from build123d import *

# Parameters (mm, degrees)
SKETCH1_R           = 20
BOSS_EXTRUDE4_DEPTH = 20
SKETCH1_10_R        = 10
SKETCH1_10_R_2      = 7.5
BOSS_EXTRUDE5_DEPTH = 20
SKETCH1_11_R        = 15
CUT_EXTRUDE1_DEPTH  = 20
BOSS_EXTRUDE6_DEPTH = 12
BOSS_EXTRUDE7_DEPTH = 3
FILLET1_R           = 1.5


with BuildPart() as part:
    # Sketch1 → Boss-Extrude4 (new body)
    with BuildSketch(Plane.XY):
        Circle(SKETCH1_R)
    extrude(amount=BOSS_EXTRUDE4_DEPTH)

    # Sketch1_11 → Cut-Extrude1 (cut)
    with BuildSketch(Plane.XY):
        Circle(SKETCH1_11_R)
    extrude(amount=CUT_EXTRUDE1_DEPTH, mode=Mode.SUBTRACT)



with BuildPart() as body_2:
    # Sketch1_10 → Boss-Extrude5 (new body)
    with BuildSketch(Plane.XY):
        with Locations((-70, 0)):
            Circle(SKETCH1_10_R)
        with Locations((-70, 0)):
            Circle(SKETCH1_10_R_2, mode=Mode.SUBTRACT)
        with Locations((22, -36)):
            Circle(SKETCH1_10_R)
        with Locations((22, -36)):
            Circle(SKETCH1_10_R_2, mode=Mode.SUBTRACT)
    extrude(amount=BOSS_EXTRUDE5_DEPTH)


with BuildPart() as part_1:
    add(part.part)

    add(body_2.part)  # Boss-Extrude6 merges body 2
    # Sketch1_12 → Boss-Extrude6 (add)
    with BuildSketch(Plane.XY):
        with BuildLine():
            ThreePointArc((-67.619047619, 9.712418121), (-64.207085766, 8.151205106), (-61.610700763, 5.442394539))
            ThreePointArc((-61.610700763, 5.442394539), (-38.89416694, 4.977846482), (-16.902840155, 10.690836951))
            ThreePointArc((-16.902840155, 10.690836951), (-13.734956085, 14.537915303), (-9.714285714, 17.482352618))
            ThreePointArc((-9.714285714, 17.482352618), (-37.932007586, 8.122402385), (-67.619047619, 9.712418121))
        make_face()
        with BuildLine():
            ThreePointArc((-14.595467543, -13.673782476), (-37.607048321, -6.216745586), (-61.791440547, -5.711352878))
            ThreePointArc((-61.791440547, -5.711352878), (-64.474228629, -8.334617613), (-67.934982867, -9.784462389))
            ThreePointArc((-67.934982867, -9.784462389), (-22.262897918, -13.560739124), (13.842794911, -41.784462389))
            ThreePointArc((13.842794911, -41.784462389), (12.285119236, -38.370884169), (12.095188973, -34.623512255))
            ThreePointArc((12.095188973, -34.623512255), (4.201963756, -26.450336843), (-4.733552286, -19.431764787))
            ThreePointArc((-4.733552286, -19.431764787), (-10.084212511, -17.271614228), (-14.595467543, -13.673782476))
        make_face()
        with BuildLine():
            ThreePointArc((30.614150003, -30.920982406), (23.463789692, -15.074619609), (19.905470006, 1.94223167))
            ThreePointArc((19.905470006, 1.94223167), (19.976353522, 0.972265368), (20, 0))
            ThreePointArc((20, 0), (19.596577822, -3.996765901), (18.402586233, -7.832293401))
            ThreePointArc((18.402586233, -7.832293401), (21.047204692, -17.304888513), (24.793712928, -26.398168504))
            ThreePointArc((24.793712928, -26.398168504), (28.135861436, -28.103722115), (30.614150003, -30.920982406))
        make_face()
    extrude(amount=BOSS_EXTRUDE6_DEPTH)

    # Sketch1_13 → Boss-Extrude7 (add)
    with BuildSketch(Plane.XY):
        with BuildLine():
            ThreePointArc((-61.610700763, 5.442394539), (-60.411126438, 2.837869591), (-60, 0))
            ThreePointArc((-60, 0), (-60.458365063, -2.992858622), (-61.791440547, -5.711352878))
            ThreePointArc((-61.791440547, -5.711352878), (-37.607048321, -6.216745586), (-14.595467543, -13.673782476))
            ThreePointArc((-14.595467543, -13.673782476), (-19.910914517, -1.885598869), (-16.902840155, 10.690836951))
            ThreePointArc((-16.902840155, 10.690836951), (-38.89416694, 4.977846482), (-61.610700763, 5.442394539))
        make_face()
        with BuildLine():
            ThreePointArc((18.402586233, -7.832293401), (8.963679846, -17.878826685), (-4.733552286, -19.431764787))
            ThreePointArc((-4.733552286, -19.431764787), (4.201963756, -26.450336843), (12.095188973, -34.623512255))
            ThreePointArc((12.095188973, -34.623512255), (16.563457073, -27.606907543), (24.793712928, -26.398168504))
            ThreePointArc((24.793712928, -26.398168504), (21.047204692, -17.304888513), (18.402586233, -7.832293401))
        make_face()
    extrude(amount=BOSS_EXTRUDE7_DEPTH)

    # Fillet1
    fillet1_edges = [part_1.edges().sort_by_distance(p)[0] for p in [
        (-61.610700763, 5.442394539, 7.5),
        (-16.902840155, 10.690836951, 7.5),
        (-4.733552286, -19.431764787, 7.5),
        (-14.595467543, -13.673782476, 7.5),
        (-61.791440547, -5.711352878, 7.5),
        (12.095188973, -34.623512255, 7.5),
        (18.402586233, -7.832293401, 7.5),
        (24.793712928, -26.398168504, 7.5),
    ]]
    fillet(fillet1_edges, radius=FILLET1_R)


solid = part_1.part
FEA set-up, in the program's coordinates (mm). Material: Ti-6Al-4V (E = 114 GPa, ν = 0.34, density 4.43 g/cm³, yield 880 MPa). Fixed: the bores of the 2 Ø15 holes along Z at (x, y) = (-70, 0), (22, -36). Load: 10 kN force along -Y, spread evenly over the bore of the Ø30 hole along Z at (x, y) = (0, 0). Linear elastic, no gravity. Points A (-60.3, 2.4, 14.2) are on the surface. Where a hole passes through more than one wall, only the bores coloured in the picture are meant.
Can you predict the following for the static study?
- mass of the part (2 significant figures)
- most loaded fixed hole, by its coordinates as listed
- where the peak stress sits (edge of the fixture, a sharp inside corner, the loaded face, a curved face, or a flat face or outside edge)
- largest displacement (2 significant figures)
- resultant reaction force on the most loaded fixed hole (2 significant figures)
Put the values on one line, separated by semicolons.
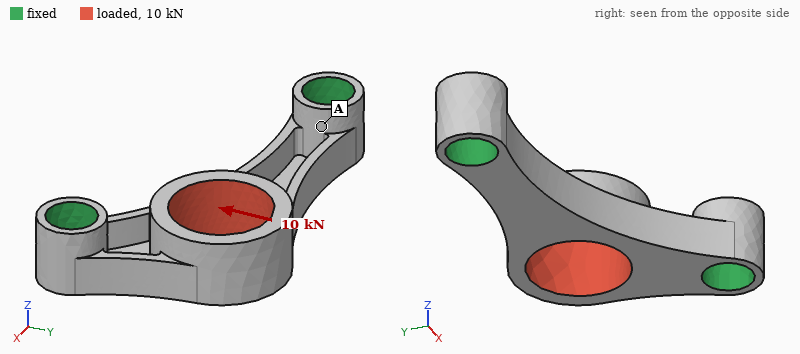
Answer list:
110 g; (22, -36); a curved face; 0.39 mm; 10 kN
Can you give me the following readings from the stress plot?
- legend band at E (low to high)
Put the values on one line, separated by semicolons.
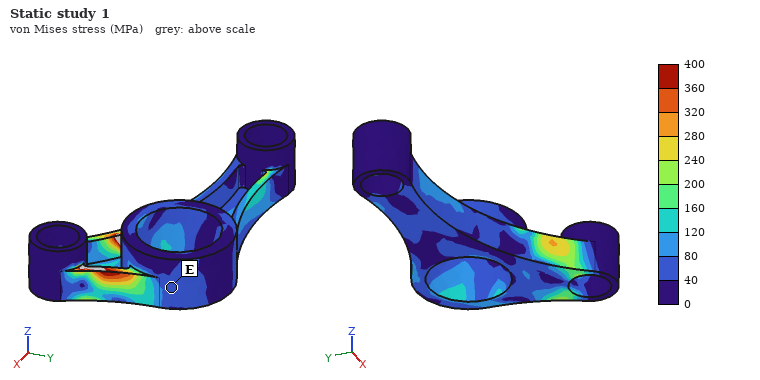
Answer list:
40 to 80 MPa
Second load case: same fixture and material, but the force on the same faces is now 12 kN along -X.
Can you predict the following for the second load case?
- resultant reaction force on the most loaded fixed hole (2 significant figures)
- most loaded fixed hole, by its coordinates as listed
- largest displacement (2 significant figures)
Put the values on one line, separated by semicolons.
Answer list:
8.8 kN; (-70, 0); 0.23 mm
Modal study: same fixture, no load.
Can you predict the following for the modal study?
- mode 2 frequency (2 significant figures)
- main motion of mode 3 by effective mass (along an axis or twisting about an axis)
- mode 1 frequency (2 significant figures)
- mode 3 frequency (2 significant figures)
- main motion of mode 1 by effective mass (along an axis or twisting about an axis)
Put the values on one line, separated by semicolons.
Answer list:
5700 Hz; along Y; 2500 Hz; 8100 Hz; along Z
